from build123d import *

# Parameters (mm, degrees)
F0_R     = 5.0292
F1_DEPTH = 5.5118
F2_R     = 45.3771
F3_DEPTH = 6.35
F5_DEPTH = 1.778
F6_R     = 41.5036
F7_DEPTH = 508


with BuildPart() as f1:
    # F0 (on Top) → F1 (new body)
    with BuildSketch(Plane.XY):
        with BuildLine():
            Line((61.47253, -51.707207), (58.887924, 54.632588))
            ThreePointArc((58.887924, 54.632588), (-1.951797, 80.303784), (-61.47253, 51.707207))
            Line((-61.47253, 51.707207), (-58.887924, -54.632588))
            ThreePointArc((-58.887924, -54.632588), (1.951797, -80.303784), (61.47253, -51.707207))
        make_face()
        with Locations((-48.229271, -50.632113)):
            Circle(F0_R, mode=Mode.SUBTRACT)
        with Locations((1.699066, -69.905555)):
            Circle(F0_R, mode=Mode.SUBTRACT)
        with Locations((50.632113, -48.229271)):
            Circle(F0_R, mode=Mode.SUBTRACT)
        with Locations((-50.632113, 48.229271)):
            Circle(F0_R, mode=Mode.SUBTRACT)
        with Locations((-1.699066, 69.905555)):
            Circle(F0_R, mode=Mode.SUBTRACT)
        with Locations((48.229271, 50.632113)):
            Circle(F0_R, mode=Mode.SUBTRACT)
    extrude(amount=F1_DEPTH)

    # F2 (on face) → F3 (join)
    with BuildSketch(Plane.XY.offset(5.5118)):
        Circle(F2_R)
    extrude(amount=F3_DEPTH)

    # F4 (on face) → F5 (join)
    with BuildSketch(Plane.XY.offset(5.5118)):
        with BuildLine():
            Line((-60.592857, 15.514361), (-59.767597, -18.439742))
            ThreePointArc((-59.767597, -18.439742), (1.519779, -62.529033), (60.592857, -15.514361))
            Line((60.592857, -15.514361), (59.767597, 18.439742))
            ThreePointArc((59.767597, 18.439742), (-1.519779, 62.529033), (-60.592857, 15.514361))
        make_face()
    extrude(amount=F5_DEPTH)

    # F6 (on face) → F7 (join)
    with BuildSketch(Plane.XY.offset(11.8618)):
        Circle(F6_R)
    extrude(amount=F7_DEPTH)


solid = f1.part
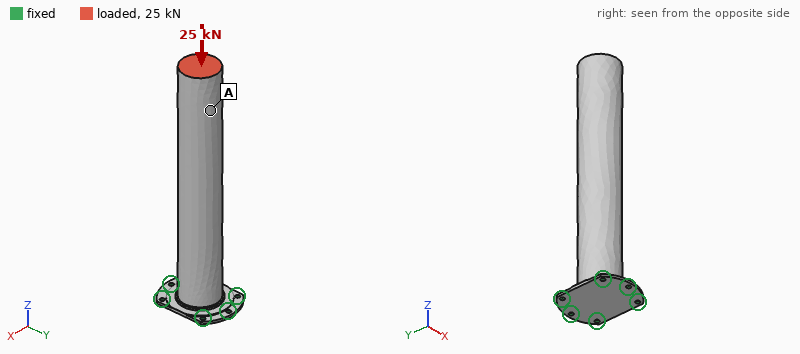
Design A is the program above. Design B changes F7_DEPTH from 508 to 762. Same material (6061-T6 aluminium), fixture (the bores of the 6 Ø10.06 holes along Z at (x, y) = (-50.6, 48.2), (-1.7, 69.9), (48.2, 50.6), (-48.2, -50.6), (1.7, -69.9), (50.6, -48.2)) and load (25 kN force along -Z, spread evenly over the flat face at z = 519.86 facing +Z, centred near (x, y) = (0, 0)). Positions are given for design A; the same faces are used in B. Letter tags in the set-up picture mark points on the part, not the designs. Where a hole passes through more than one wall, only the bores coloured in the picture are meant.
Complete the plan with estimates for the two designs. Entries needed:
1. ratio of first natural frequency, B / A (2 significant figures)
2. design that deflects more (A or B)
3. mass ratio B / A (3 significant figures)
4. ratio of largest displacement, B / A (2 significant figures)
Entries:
0.53
B
1.48
1.1
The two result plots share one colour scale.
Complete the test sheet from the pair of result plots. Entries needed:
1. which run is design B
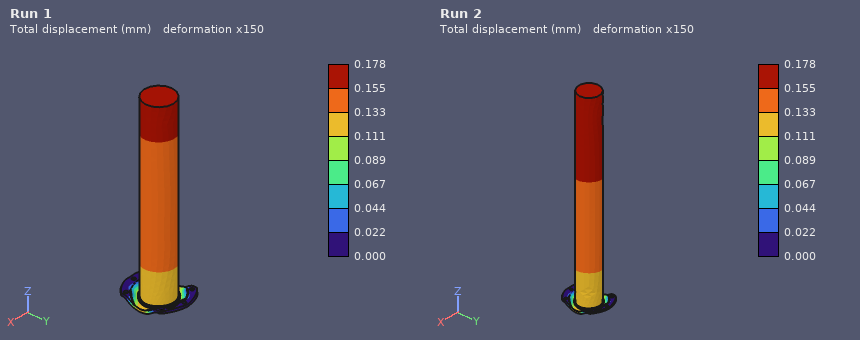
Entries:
Run 2
